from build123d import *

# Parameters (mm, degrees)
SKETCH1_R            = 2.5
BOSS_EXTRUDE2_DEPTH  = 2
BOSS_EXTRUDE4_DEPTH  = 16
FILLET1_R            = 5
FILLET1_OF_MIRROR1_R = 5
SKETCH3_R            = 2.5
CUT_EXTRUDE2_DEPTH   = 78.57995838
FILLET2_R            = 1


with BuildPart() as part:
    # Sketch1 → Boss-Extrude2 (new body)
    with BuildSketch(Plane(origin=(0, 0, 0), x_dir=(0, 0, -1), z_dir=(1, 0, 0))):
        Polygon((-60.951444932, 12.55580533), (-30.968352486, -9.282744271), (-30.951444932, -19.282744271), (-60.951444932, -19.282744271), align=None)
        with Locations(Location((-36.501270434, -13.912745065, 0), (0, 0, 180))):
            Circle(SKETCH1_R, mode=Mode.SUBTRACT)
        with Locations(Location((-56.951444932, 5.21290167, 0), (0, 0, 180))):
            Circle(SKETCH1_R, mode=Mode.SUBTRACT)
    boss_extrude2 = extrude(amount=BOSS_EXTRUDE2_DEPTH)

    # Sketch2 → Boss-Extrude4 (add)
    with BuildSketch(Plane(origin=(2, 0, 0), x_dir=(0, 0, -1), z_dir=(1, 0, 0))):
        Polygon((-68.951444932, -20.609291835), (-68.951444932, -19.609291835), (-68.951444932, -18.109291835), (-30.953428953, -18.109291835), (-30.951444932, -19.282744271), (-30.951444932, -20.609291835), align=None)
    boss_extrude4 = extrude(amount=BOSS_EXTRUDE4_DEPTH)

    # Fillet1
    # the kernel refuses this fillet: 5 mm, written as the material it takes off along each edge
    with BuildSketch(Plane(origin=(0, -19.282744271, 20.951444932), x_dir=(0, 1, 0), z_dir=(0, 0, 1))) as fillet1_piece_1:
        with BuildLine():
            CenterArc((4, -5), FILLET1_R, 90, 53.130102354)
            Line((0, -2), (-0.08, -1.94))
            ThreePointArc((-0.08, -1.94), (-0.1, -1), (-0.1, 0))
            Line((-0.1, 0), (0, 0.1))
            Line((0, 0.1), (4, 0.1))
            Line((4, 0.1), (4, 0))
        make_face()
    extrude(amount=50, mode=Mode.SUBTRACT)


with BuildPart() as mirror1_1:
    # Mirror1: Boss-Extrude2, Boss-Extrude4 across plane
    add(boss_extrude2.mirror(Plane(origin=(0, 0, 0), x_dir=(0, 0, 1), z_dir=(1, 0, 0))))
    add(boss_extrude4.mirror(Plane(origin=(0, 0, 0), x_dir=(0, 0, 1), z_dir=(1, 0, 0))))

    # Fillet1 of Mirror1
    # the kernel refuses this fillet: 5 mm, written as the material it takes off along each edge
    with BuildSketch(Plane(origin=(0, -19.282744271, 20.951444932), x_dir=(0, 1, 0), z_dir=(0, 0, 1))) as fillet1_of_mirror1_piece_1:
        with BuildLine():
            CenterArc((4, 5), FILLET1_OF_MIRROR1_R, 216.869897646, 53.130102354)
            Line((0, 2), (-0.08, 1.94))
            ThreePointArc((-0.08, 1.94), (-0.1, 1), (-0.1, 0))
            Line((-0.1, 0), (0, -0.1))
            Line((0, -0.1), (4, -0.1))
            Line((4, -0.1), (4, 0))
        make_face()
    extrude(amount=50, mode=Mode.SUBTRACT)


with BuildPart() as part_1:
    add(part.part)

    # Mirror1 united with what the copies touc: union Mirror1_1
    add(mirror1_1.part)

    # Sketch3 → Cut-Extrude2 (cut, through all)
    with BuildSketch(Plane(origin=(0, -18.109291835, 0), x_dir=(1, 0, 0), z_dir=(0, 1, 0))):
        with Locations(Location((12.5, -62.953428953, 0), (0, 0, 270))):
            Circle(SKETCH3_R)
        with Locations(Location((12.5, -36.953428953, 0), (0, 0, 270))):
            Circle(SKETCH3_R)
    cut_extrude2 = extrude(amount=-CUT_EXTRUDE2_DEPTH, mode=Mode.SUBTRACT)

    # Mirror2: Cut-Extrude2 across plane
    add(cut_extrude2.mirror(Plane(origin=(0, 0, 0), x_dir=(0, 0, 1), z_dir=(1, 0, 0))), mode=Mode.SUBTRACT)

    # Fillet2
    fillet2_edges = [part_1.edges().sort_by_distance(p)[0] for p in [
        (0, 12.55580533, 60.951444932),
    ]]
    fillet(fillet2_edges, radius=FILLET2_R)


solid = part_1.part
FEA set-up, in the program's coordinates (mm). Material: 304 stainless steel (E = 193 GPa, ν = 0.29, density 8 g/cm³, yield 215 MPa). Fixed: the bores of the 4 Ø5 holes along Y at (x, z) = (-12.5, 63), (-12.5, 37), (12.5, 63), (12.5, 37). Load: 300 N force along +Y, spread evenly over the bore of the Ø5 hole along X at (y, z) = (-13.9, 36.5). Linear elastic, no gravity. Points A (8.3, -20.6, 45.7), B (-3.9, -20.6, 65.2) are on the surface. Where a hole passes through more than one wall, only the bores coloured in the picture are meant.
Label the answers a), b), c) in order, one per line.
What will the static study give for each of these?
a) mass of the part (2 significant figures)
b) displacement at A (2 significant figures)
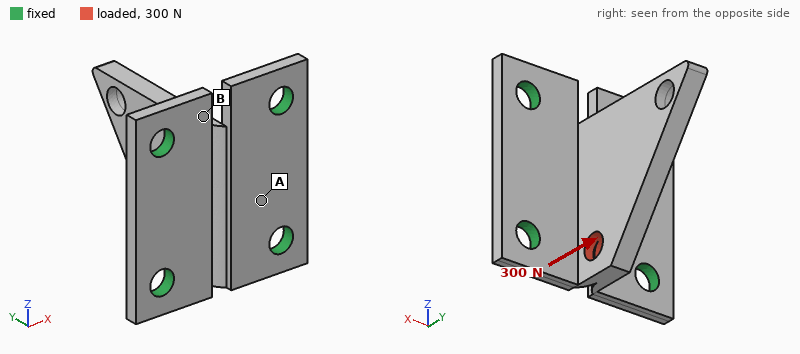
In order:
a) 40 g
b) 1.6 µm
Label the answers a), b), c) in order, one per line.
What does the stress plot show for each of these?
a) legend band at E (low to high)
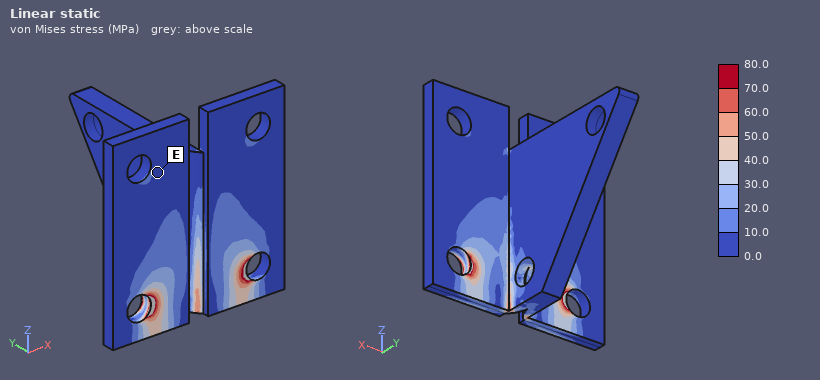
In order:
a) 0.0 to 10.0 MPa
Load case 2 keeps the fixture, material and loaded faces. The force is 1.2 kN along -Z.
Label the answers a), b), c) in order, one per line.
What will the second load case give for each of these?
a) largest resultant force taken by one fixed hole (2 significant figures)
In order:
a) 430 N
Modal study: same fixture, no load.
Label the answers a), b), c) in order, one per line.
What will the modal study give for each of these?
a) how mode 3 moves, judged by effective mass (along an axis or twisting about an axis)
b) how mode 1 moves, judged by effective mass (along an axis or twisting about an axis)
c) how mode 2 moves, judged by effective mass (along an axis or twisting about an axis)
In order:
a) along Y
b) along X
c) along Z
